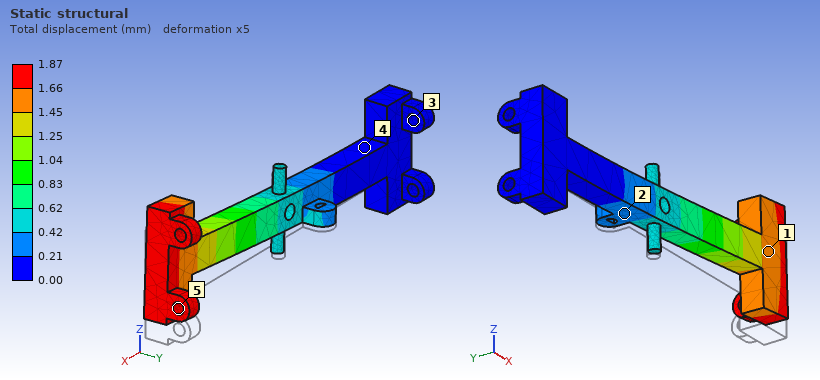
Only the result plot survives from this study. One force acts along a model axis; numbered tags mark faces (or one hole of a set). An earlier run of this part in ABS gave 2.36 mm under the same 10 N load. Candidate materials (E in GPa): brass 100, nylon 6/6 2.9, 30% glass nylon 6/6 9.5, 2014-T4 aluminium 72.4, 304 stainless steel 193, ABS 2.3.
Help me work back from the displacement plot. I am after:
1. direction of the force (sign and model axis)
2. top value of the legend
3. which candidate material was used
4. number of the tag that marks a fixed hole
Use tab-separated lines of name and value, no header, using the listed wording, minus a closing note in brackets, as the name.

direction of the force	+Z
top value of the legend	1.87 mm
which candidate material was used	nylon 6/6
number of the tag that marks a fixed hole	3
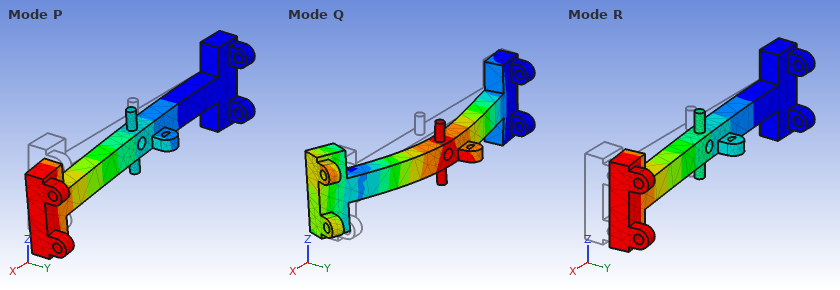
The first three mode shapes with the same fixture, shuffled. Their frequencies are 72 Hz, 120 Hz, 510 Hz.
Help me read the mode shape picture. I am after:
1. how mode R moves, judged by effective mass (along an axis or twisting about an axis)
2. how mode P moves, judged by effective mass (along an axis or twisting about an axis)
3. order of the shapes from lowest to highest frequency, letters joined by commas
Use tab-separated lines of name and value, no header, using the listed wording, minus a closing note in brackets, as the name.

how mode R moves, judged by effective mass	along Y
how mode P moves, judged by effective mass	along Z
order of the shapes from lowest to highest frequency, letters joined by commas	R, P, Q
